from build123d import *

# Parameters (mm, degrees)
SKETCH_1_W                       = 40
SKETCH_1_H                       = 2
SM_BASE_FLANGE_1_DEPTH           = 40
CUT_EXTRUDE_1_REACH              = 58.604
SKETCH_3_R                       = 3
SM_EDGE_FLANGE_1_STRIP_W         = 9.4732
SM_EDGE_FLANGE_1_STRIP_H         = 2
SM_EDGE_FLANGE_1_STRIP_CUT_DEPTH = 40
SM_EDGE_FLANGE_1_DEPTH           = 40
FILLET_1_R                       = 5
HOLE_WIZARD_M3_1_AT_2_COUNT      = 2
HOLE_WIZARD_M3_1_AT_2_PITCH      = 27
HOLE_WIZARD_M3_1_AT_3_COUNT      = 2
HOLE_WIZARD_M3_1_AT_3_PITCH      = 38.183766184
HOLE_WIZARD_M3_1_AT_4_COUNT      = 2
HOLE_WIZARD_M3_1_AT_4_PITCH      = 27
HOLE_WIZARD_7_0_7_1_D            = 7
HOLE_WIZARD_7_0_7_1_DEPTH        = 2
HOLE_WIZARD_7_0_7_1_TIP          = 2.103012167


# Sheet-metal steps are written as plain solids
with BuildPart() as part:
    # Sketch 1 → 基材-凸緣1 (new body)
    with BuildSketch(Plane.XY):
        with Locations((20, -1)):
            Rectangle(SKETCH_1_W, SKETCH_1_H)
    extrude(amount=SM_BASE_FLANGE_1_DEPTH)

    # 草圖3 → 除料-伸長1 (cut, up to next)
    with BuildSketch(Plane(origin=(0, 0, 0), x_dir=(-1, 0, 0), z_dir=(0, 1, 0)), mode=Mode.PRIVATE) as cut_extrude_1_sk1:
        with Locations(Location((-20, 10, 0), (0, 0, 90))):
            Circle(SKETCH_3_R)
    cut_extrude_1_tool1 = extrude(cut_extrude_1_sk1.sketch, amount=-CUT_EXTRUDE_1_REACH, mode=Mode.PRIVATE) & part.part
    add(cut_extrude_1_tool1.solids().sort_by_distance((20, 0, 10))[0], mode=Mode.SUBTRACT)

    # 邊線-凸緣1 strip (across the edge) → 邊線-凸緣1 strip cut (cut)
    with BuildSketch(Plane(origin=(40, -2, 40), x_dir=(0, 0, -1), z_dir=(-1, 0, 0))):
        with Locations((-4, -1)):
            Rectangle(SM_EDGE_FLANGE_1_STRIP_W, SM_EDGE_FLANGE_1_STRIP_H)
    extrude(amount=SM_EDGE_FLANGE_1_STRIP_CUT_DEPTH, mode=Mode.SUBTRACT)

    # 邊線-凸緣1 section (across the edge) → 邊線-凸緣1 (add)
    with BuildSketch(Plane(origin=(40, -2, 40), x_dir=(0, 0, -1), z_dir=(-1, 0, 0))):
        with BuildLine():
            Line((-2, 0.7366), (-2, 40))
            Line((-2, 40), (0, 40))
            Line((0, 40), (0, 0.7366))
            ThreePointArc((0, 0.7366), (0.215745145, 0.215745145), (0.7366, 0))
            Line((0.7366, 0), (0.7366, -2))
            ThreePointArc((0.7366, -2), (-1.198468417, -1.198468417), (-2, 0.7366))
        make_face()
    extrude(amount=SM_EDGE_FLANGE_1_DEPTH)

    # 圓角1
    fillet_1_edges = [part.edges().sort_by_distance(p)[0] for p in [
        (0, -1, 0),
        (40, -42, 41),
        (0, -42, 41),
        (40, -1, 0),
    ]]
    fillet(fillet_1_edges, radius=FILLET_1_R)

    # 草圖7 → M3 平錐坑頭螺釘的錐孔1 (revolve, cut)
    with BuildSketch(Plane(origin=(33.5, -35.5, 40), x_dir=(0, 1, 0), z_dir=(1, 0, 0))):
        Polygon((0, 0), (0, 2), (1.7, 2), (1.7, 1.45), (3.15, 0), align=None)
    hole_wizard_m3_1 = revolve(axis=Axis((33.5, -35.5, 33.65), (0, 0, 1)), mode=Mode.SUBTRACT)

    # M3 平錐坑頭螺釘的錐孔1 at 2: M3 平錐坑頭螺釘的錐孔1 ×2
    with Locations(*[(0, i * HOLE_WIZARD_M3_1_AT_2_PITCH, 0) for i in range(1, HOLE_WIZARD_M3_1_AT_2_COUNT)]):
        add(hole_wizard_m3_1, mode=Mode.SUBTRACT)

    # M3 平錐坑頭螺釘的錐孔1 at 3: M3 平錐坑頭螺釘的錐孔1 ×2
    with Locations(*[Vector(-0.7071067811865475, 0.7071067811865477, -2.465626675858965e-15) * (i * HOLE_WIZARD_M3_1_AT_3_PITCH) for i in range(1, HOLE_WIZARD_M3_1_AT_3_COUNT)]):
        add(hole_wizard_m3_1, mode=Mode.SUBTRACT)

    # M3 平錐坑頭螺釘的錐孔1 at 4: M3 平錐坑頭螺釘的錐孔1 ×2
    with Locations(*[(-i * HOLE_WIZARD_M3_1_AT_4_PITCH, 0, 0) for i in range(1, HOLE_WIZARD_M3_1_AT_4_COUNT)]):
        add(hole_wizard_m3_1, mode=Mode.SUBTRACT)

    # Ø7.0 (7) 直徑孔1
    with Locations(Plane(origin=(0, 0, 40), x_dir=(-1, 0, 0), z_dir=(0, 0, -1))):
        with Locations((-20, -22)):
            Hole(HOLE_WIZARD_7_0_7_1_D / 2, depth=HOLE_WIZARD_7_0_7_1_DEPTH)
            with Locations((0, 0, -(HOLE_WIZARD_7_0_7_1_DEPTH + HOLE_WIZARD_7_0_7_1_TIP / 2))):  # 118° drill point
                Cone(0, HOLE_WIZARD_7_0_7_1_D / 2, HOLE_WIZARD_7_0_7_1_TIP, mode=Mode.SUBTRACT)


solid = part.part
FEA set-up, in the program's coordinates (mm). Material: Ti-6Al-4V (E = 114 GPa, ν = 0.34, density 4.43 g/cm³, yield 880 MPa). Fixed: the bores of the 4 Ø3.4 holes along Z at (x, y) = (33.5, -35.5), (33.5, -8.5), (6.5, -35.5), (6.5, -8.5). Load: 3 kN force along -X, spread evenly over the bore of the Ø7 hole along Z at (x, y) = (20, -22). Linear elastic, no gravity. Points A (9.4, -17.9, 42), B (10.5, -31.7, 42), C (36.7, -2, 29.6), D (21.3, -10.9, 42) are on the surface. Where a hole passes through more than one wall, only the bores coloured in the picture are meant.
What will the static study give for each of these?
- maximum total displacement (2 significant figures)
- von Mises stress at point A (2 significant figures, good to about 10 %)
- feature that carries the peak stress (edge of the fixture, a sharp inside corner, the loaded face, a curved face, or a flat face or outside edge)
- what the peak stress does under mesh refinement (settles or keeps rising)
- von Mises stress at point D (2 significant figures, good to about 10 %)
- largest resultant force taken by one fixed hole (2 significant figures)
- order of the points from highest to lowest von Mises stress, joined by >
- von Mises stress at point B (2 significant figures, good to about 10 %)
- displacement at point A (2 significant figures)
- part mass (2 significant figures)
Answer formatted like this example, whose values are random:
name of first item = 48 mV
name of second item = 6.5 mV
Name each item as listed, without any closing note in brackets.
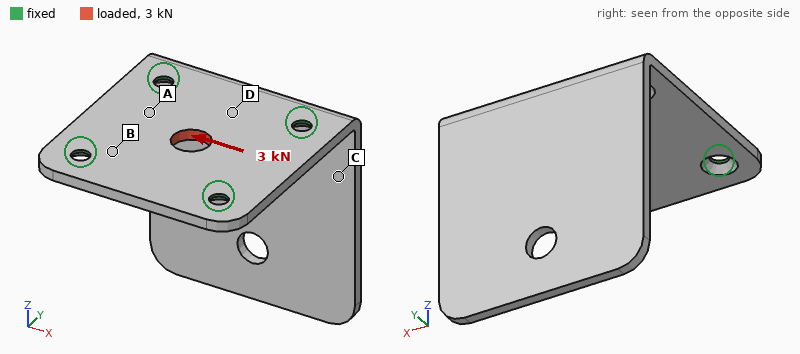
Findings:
maximum total displacement = 10 µm
von Mises stress at point A = 40 MPa
feature that carries the peak stress = edge of the fixture
what the peak stress does under mesh refinement = keeps rising
von Mises stress at point D = 29 MPa
largest resultant force taken by one fixed hole = 800 N
order of the points from highest to lowest von Mises stress, joined by > = B > A > D > C
von Mises stress at point B = 60 MPa
displacement at point A = 6.5 µm
part mass = 27 g
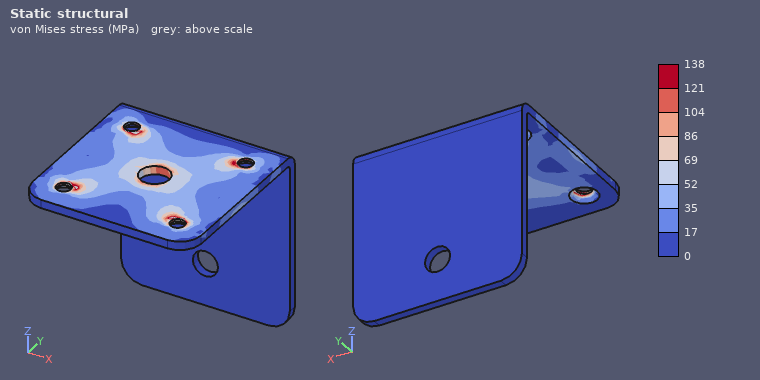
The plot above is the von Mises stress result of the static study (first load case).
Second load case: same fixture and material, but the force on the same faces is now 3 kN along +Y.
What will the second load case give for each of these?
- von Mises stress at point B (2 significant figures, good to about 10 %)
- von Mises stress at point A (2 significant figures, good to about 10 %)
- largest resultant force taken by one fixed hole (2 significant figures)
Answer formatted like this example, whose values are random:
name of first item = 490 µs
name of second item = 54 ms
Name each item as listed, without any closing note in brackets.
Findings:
von Mises stress at point B = 58 MPa
von Mises stress at point A = 32 MPa
largest resultant force taken by one fixed hole = 800 N
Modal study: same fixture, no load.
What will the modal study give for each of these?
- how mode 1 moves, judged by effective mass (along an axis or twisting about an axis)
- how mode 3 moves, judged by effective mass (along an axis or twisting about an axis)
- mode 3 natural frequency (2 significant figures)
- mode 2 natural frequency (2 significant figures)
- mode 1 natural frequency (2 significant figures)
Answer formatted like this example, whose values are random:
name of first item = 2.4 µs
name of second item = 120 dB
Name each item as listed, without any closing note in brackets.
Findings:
how mode 1 moves, judged by effective mass = along Y
how mode 3 moves, judged by effective mass = along X
mode 3 natural frequency = 3200 Hz
mode 2 natural frequency = 2000 Hz
mode 1 natural frequency = 730 Hz
